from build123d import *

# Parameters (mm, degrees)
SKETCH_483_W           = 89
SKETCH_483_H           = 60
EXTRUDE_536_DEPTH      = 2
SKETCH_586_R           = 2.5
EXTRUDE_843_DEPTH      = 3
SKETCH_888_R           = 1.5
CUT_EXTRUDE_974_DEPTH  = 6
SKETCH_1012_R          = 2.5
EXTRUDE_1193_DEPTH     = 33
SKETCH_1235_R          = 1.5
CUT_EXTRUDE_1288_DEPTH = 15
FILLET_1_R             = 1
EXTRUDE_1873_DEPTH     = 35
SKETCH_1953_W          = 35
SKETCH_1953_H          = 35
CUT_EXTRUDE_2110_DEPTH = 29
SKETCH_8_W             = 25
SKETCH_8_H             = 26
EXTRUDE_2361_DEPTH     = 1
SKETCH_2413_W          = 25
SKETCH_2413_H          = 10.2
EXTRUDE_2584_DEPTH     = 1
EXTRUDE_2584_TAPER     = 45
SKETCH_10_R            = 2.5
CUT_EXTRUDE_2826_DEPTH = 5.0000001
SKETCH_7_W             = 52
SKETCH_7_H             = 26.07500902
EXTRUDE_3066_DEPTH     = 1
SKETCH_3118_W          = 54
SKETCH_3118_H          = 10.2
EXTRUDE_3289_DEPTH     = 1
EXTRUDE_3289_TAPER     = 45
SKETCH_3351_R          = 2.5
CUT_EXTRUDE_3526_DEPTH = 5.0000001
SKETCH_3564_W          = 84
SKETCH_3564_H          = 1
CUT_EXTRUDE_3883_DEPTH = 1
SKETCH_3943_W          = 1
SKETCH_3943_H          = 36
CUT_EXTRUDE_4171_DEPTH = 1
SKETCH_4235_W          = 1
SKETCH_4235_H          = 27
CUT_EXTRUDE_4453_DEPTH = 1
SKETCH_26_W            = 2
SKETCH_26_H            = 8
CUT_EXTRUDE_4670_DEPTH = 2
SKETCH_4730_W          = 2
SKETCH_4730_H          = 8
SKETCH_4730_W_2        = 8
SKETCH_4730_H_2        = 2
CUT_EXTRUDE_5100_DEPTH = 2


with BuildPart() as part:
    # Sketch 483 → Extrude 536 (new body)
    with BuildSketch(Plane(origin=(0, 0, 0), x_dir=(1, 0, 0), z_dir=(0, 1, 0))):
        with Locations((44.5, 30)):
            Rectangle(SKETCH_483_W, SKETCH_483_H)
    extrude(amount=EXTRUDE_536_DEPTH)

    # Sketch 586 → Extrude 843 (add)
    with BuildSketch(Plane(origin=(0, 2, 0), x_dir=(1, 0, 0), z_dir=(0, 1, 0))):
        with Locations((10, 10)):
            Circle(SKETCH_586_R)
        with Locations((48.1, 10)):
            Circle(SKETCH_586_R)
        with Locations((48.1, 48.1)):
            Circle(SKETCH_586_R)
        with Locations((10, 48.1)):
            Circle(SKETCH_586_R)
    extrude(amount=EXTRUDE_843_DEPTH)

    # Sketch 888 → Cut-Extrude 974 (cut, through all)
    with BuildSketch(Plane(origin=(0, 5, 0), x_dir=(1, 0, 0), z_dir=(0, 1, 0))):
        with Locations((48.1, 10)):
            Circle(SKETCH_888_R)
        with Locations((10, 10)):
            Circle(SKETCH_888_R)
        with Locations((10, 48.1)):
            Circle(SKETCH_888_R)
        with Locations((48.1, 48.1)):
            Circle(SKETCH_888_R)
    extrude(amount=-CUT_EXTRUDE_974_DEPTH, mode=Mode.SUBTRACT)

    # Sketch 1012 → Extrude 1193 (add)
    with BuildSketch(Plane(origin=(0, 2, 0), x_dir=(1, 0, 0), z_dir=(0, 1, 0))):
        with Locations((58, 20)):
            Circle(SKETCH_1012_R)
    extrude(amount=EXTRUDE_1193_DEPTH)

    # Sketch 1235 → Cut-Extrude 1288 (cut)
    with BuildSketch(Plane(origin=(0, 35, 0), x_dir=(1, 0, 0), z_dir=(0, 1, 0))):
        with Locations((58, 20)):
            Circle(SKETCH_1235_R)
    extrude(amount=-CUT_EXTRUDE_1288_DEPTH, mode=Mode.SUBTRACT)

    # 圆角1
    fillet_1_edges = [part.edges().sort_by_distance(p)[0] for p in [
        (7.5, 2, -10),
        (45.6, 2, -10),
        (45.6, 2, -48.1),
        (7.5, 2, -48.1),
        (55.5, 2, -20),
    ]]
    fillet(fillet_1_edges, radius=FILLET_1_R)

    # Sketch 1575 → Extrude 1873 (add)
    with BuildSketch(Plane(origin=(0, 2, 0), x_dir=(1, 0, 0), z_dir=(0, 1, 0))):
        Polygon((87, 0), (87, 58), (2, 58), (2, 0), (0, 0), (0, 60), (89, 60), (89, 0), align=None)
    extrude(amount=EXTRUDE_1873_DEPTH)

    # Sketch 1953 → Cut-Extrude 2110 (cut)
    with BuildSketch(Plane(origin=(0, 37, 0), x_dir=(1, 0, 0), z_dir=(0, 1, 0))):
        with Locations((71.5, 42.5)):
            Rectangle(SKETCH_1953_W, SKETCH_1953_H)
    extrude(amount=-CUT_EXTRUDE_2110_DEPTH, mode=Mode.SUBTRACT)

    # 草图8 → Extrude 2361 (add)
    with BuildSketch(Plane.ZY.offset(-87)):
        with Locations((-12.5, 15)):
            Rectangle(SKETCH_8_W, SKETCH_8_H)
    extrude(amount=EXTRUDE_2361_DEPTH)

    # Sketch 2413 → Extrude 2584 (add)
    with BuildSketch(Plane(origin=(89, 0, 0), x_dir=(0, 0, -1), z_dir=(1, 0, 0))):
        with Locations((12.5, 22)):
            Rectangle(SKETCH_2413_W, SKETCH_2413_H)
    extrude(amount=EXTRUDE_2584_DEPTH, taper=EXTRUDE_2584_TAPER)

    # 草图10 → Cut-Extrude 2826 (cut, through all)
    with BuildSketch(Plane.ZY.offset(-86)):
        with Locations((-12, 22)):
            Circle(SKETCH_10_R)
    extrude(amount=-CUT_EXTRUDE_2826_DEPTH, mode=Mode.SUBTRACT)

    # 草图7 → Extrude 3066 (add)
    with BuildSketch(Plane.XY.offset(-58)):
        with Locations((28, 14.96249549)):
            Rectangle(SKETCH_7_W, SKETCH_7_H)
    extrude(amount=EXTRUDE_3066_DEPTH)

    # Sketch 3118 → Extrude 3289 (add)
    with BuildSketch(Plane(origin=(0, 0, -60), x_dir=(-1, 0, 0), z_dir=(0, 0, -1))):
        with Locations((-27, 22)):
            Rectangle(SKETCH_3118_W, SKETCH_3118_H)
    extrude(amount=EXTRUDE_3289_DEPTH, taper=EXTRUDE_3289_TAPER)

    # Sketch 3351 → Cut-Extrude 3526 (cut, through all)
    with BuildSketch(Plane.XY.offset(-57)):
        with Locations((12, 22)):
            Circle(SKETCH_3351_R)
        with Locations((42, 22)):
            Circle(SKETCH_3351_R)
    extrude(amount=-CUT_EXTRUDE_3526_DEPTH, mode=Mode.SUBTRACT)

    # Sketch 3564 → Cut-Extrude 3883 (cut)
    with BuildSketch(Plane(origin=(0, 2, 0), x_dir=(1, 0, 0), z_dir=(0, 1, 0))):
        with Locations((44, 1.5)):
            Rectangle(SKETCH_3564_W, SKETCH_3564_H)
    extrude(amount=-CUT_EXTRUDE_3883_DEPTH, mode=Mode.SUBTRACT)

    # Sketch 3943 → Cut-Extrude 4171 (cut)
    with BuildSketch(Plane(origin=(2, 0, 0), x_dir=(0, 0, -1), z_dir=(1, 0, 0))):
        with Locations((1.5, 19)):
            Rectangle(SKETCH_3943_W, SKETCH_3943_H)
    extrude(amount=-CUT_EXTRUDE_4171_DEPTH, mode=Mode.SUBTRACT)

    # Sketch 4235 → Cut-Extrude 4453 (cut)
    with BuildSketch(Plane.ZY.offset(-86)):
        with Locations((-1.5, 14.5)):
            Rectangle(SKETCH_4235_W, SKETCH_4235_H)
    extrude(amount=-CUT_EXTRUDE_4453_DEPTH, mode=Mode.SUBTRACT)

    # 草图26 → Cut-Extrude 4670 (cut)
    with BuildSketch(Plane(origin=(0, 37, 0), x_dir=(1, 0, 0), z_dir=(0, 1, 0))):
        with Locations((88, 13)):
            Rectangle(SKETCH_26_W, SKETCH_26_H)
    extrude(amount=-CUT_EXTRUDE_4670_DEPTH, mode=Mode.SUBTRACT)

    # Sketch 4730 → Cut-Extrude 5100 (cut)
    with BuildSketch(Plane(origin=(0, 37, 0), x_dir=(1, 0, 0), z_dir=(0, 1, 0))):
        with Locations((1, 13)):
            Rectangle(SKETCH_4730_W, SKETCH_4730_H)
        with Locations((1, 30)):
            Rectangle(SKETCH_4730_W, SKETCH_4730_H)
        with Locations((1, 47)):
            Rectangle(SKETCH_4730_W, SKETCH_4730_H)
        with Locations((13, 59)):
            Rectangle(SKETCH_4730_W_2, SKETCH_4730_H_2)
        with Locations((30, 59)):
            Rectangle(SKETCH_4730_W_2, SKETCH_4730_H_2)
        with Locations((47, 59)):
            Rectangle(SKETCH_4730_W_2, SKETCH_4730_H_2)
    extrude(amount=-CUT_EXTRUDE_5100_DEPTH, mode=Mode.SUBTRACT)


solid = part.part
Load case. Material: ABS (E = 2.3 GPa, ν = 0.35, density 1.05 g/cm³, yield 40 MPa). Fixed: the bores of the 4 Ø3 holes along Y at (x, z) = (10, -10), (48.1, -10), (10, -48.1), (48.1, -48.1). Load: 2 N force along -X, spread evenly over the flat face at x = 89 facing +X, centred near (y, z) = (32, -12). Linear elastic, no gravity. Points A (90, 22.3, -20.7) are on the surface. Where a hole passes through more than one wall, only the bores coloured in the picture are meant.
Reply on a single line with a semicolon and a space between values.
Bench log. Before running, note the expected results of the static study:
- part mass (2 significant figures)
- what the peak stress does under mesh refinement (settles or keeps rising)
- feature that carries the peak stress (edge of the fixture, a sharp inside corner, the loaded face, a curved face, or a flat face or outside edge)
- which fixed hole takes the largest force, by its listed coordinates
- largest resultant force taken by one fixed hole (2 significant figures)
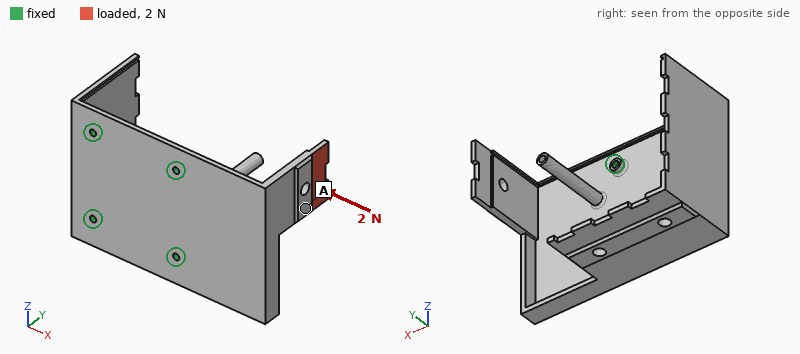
25 g; keeps rising; a sharp inside corner; (48.1, -10); 2.5 N
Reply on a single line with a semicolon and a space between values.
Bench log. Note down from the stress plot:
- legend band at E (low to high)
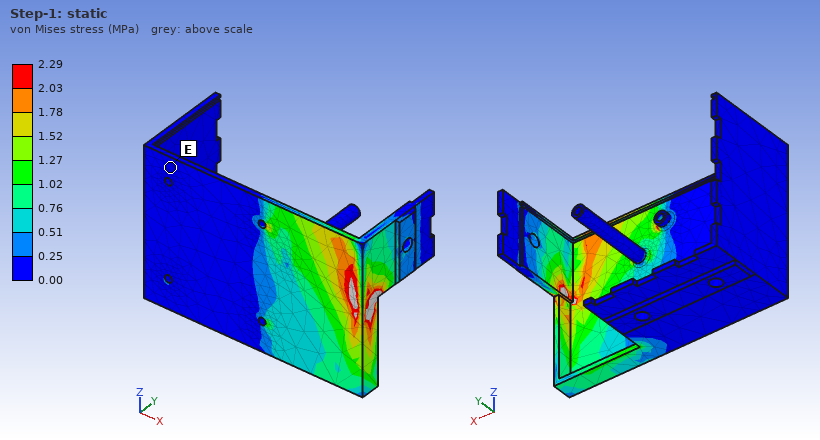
0.00 to 0.25 MPa
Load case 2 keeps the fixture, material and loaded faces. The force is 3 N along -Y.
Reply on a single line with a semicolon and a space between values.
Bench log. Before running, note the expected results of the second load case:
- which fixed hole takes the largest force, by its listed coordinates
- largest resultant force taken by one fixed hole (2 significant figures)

(48.1, -10); 3.4 N
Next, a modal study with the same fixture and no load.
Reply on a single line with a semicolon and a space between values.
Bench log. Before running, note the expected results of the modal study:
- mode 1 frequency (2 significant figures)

160 Hz
